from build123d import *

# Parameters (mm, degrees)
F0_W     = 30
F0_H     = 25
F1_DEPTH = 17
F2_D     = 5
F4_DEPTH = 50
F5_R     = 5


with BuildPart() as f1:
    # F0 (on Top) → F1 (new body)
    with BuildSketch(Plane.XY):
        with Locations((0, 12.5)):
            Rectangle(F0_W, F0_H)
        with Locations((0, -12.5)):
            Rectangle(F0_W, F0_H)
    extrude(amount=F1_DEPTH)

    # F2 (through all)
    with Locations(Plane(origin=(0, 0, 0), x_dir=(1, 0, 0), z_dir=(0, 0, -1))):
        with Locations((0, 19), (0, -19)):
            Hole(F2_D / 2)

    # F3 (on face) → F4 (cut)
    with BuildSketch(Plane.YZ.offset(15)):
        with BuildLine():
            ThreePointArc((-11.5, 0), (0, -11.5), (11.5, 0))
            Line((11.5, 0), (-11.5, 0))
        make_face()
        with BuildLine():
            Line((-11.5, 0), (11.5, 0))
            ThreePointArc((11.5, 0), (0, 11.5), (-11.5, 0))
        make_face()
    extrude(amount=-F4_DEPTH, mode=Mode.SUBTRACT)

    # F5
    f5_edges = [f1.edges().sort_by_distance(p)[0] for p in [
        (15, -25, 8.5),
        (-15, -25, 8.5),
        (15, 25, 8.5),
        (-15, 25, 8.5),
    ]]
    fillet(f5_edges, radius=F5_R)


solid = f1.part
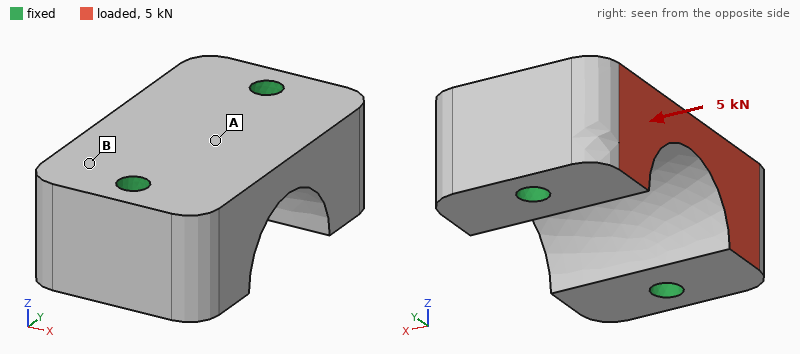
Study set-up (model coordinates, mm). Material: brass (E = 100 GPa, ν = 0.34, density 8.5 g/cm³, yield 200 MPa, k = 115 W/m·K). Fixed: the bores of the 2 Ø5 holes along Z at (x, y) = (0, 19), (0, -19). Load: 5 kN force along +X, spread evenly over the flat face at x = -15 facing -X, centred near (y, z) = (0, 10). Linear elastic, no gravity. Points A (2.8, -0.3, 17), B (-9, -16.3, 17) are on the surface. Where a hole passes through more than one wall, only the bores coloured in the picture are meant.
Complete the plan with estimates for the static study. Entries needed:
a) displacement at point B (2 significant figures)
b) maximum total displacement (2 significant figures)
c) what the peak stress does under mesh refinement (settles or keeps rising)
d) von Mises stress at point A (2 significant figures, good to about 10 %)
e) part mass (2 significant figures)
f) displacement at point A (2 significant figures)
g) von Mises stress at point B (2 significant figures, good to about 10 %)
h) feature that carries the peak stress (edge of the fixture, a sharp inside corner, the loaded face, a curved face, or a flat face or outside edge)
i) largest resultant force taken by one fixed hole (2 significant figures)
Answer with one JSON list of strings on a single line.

["1.5 µm", "4.9 µm", "keeps rising", "5.1 MPa", "160 g", "3.1 µm", "14 MPa", "edge of the fixture", "2.5 kN"]
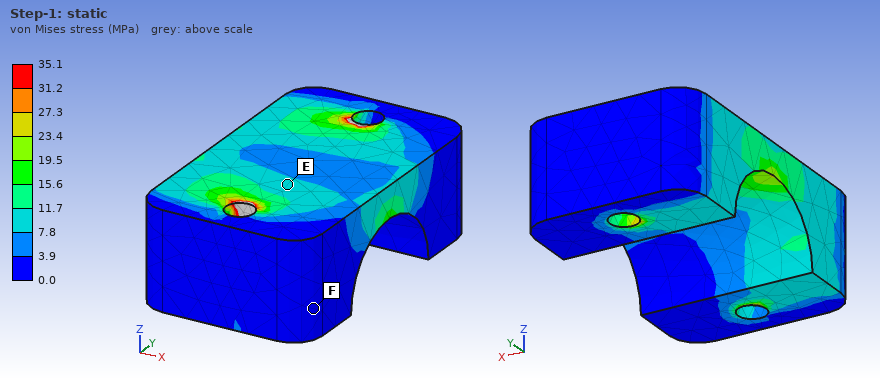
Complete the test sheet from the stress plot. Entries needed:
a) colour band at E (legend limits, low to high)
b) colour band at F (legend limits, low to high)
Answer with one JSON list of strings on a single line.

["7.8 to 11.7 MPa", "0.0 to 3.9 MPa"]
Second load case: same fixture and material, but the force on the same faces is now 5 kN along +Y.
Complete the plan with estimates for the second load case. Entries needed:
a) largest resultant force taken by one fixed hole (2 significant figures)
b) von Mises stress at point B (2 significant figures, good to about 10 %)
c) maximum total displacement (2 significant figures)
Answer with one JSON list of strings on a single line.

["2.9 kN", "17 MPa", "8.1 µm"]
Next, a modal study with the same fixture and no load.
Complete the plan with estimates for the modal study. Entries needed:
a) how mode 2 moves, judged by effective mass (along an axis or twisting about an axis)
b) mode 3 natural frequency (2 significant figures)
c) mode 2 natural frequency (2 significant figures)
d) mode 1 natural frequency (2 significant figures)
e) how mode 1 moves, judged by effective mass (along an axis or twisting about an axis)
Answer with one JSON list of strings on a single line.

["along Z", "23 kHz", "20 kHz", "17 kHz", "along X"]
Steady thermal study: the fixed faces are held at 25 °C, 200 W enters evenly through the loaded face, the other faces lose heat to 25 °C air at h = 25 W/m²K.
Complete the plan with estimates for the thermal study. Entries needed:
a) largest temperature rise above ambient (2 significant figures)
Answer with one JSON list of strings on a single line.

["59 K"]
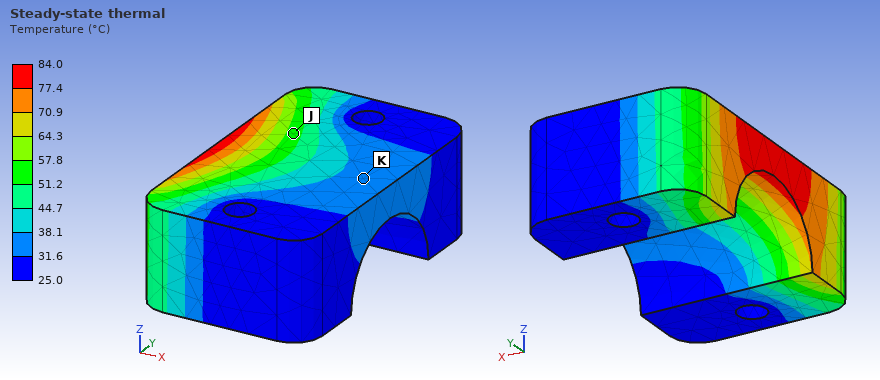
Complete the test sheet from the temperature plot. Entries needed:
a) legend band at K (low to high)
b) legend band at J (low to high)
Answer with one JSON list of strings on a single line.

["31.6 to 38.1 °C", "51.2 to 57.8 °C"]
